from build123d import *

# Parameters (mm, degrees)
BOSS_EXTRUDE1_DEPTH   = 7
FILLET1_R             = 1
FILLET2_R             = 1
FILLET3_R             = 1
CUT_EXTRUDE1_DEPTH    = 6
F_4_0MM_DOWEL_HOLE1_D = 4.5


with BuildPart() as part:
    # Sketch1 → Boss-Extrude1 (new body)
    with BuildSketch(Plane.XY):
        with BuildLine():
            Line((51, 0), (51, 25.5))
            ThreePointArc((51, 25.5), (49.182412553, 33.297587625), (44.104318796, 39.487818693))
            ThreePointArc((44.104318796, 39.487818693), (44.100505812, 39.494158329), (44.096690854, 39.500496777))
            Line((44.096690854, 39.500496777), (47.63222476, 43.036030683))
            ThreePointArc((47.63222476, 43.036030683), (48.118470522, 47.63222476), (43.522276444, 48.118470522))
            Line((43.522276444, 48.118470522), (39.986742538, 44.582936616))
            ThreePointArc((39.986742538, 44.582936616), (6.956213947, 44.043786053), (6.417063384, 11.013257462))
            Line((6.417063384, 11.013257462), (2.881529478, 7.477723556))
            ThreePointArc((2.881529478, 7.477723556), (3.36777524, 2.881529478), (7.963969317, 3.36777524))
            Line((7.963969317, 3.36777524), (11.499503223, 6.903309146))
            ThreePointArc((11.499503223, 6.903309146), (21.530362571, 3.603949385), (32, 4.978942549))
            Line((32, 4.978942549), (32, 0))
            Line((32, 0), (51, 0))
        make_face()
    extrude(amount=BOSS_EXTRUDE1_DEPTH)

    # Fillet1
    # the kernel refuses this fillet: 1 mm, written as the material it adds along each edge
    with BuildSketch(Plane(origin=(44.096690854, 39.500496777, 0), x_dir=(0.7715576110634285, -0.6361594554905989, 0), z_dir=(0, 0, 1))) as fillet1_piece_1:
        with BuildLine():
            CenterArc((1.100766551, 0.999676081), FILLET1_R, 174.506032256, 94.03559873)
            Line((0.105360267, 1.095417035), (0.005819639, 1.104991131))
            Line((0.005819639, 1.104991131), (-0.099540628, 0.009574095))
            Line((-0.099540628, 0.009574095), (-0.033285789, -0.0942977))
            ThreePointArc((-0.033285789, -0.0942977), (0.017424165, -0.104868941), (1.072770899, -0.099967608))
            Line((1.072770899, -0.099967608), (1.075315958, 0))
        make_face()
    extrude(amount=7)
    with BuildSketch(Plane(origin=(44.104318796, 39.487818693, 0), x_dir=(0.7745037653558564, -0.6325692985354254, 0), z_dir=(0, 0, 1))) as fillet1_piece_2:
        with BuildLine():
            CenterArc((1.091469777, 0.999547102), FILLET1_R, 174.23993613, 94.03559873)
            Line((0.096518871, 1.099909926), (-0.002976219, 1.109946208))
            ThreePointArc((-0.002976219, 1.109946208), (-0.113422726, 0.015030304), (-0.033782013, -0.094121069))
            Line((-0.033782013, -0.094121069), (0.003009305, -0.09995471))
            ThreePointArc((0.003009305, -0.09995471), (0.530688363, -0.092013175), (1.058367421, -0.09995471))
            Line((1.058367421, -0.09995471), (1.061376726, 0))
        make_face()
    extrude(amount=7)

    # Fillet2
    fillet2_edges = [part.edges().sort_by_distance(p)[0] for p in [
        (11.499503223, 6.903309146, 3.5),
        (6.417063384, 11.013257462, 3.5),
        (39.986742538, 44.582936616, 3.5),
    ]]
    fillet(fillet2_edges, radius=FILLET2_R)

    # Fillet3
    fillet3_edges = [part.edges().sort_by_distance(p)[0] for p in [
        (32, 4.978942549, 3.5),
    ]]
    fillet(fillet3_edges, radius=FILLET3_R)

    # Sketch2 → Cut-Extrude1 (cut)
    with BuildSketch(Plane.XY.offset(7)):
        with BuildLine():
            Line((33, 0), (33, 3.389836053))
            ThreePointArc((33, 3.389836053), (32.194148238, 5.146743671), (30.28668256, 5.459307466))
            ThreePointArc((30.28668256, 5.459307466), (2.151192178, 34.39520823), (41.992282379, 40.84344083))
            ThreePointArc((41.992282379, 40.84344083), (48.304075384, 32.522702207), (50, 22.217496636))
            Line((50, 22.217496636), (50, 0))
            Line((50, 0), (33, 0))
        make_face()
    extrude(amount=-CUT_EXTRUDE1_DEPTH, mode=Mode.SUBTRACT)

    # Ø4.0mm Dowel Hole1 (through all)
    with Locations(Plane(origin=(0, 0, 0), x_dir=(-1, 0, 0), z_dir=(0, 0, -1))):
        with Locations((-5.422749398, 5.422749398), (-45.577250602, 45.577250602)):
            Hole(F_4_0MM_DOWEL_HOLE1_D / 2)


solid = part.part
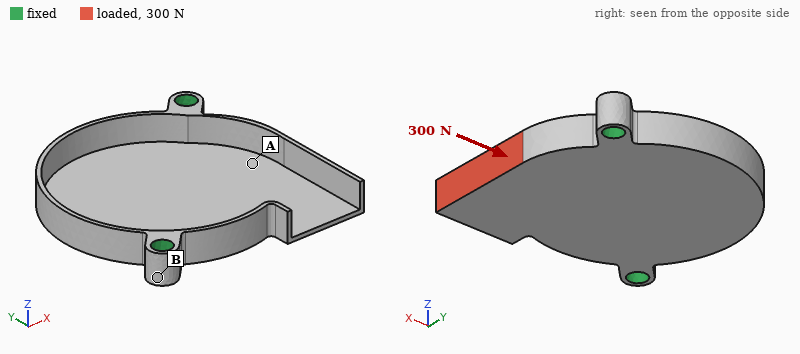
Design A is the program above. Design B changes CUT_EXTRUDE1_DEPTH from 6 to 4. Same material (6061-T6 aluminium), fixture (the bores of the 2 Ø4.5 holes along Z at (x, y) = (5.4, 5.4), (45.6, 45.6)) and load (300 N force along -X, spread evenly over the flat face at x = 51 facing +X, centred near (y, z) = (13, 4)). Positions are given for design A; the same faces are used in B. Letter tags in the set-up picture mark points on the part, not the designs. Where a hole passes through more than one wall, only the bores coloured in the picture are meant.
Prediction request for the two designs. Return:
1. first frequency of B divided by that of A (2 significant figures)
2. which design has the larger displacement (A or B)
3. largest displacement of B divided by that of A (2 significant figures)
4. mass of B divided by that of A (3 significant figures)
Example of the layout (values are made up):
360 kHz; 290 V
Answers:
1.2; A; 0.11; 2.12
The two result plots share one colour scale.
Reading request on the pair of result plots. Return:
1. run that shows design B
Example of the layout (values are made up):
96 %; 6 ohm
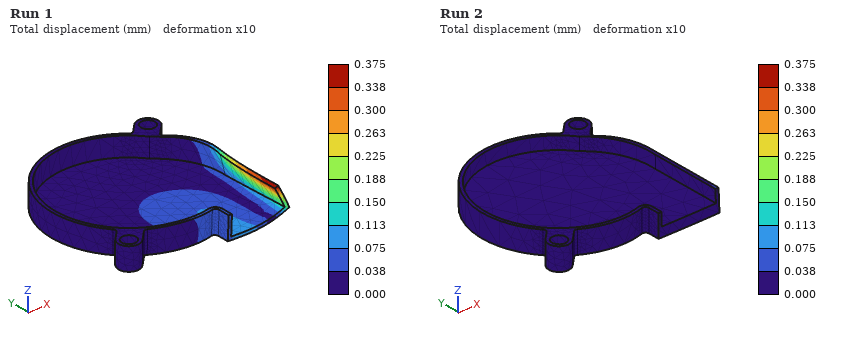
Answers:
Run 2
